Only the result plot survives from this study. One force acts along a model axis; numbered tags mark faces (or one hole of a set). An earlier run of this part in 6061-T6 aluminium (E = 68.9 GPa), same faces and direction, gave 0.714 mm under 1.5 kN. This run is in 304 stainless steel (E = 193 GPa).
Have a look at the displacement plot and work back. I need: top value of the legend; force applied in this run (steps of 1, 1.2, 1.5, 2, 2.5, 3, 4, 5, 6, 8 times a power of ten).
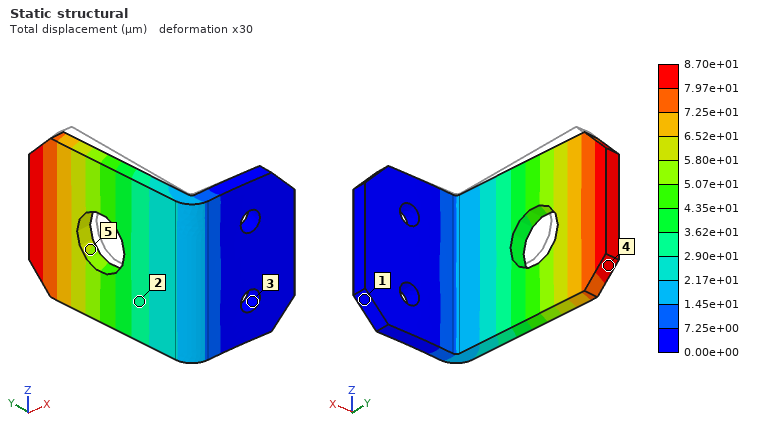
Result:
8.70e+01 µm
500 N
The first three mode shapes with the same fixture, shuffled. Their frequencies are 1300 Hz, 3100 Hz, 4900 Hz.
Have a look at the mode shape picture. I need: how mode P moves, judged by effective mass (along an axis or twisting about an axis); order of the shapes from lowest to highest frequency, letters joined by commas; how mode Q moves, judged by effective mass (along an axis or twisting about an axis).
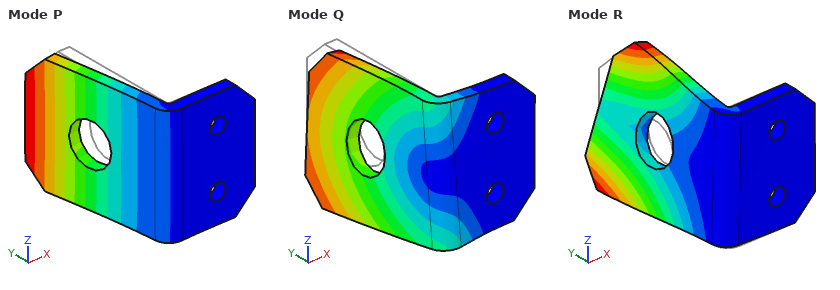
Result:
along X
P, Q, R
along Z
